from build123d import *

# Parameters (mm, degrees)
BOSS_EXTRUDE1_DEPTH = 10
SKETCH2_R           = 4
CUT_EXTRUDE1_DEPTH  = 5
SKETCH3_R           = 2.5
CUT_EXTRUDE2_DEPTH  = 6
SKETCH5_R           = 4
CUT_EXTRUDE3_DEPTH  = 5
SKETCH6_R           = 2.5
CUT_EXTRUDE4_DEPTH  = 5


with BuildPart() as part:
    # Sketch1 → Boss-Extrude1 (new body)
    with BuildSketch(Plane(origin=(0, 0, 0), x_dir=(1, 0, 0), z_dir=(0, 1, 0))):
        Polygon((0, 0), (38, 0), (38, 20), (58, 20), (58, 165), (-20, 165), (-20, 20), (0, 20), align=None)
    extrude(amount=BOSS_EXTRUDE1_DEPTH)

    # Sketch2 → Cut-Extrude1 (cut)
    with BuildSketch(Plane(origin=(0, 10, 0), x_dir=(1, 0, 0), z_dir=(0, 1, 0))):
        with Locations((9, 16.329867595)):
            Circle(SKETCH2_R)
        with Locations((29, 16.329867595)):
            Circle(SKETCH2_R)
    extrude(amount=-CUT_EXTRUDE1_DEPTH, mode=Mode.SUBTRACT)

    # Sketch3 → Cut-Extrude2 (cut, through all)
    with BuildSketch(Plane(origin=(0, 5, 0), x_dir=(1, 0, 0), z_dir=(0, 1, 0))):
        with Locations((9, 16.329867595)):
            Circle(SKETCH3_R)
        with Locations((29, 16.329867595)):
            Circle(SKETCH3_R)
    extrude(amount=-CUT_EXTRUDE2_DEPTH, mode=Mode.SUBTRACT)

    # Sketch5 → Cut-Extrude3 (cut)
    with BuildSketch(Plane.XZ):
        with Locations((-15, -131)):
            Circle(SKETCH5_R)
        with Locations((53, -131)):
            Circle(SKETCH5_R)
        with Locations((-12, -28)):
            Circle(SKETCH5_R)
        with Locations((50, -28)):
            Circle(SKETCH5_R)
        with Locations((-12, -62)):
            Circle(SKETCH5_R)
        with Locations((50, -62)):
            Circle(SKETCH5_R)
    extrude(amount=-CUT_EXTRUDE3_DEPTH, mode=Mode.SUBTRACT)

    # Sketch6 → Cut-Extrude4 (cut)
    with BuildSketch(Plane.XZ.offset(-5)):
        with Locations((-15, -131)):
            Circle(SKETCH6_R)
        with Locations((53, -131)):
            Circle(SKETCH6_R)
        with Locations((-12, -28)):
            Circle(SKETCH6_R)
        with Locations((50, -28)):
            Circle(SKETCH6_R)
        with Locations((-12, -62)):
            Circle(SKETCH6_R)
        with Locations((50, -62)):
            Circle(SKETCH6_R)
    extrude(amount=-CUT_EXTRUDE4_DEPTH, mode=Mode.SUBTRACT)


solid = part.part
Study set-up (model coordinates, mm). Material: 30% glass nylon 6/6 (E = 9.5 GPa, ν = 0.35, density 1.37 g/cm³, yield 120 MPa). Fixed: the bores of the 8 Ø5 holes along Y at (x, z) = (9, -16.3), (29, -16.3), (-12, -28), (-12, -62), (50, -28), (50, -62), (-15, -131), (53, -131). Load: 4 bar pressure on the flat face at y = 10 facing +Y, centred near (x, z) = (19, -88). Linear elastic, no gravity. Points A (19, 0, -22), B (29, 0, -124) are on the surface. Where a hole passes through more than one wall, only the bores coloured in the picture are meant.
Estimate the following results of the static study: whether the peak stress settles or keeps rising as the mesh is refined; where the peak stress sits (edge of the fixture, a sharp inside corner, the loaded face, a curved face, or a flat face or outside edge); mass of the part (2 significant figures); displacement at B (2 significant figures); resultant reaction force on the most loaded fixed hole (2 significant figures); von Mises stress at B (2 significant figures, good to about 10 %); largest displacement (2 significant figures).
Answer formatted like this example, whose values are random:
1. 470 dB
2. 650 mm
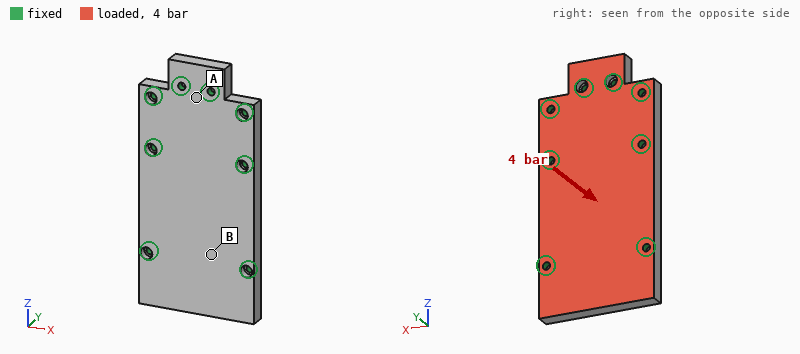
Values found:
1. keeps rising
2. edge of the fixture
3. 160 g
4. 0.096 mm
5. 1.3 kN
6. 12 MPa
7. 0.27 mm
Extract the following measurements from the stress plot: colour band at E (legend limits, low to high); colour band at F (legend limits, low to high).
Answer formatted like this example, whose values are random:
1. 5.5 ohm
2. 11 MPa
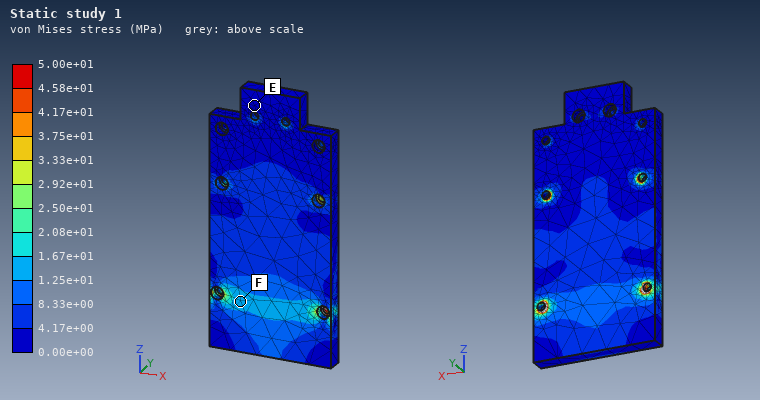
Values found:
1. 0.00e+00 to 4.17e+00 MPa
2. 1.25e+01 to 1.67e+01 MPa
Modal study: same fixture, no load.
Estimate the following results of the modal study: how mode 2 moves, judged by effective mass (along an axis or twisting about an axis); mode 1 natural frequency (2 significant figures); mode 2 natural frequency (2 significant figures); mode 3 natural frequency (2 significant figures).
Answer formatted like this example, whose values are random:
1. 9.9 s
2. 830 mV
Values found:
1. along Y
2. 2000 Hz
3. 3100 Hz
4. 3800 Hz
